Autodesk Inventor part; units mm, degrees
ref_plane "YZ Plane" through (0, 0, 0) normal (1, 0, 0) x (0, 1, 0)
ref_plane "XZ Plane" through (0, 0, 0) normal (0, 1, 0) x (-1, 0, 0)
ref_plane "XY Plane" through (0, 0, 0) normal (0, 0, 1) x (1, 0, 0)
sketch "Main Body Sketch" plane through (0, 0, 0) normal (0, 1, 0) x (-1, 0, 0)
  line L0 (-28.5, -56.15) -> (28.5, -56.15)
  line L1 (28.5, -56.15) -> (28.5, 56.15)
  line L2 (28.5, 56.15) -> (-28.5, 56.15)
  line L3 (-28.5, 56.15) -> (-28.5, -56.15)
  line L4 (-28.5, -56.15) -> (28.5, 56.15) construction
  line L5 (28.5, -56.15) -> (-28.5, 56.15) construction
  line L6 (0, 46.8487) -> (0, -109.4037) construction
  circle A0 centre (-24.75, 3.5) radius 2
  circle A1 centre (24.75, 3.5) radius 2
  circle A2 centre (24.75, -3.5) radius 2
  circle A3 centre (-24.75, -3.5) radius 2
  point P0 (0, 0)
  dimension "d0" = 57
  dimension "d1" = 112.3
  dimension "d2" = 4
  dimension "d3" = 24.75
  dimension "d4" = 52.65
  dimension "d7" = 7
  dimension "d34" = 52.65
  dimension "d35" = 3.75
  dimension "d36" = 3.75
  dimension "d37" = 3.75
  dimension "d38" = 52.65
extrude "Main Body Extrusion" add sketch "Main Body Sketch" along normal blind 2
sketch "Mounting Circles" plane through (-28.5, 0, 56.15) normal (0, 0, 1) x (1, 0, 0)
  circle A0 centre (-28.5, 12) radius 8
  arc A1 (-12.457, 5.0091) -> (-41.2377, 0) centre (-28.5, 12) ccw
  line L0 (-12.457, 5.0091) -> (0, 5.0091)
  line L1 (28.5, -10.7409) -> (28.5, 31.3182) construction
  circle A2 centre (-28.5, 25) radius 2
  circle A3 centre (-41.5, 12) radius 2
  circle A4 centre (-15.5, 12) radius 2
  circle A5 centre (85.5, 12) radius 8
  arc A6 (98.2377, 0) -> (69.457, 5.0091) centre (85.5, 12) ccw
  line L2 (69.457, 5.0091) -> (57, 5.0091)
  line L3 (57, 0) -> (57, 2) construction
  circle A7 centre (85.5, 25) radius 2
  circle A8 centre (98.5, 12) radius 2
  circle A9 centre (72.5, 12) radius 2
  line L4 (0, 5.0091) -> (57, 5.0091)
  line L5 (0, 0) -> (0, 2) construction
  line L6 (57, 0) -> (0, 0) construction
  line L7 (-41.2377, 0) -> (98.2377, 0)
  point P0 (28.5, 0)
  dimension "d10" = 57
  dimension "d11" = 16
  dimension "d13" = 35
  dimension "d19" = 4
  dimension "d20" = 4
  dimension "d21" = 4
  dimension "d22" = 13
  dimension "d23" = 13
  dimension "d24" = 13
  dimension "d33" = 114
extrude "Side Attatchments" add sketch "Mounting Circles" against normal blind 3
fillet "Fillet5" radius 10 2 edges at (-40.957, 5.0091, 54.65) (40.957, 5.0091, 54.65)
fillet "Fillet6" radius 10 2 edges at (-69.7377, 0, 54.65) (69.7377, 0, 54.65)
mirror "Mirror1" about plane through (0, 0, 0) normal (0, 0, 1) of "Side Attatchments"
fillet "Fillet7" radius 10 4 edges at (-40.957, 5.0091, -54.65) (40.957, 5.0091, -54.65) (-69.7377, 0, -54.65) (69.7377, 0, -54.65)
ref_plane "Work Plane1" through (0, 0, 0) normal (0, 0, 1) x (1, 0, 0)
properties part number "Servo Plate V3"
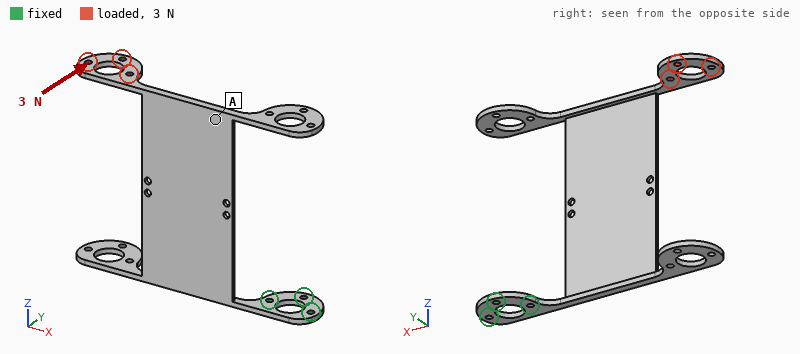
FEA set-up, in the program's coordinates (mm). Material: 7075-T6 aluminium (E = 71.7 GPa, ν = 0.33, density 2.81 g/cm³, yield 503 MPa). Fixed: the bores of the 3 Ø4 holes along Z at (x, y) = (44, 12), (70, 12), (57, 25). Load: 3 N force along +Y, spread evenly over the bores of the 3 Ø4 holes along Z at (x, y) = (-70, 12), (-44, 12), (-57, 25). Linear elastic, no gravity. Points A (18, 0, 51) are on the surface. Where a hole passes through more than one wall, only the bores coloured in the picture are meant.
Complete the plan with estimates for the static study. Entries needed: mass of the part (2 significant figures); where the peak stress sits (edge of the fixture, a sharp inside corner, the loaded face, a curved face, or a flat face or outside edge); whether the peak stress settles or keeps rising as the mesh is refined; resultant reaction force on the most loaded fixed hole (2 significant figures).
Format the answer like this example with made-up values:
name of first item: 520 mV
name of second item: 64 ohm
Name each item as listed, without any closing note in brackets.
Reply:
mass of the part: 63 g
where the peak stress sits: a sharp inside corner
whether the peak stress settles or keeps rising as the mesh is refined: keeps rising
resultant reaction force on the most loaded fixed hole: 13 N
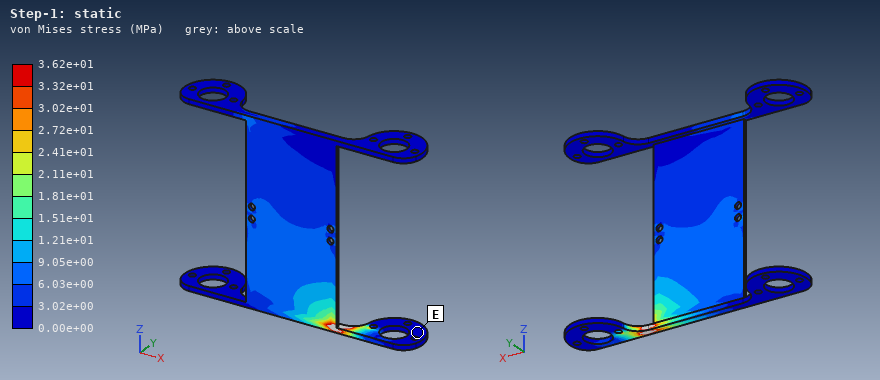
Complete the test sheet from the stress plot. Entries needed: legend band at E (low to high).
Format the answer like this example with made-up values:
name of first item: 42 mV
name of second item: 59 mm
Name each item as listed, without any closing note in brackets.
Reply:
legend band at E: 0.00e+00 to 3.02e+00 MPa
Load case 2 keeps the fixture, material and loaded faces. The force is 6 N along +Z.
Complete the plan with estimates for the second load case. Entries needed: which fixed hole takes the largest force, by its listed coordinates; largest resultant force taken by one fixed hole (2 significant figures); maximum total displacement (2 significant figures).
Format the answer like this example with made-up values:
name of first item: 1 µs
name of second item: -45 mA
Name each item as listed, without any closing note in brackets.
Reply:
which fixed hole takes the largest force, by its listed coordinates: (44, 12)
largest resultant force taken by one fixed hole: 12 N
maximum total displacement: 1.7 mm
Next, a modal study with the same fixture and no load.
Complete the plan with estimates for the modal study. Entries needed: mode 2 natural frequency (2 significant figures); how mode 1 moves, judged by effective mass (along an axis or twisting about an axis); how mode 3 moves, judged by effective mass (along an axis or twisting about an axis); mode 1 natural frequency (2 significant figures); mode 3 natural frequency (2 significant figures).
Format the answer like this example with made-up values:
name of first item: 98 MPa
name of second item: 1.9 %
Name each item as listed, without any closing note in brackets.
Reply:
mode 2 natural frequency: 56 Hz
how mode 1 moves, judged by effective mass: along Y
how mode 3 moves, judged by effective mass: twisting about Z
mode 1 natural frequency: 46 Hz
mode 3 natural frequency: 120 Hz
